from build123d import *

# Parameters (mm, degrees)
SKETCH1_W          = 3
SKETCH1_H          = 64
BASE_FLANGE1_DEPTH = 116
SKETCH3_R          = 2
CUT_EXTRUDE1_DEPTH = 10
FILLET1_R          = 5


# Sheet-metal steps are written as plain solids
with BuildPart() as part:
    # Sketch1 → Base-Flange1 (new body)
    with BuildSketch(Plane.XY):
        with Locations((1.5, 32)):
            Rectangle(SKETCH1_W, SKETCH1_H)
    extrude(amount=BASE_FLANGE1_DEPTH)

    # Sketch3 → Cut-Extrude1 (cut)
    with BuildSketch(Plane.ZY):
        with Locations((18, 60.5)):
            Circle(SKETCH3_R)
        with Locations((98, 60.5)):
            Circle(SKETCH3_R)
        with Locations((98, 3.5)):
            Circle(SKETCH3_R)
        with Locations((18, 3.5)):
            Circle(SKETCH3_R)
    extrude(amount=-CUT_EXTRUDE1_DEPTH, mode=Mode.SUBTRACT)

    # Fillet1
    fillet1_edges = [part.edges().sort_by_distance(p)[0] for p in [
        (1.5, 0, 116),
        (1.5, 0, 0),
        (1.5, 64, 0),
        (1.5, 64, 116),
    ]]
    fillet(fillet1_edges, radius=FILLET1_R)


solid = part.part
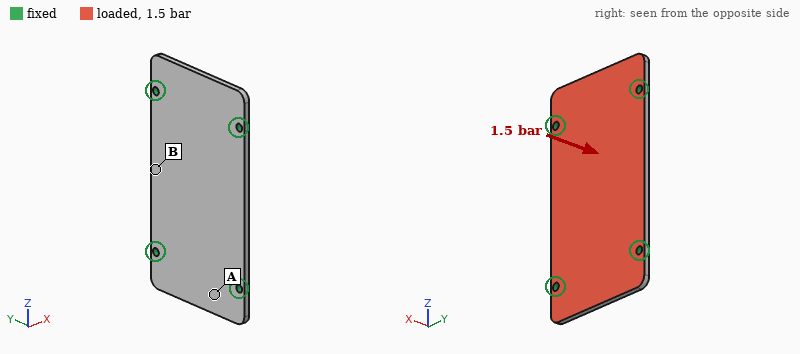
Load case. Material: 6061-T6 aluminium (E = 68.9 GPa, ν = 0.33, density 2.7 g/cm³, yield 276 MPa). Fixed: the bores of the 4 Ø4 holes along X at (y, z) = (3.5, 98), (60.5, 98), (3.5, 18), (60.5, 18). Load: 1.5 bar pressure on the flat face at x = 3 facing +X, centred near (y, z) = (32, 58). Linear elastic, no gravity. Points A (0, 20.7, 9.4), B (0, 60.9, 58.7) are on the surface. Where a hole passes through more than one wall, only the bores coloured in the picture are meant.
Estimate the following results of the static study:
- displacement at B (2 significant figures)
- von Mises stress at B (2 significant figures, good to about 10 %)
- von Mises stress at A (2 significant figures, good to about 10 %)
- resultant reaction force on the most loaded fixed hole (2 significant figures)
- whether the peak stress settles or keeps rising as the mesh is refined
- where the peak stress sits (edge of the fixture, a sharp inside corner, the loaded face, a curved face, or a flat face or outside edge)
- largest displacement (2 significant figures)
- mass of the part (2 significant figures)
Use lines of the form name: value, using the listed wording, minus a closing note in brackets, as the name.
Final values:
displacement at B: 0.13 mm
von Mises stress at B: 33 MPa
von Mises stress at A: 14 MPa
resultant reaction force on the most loaded fixed hole: 280 N
whether the peak stress settles or keeps rising as the mesh is refined: keeps rising
where the peak stress sits: edge of the fixture
largest displacement: 0.15 mm
mass of the part: 60 g
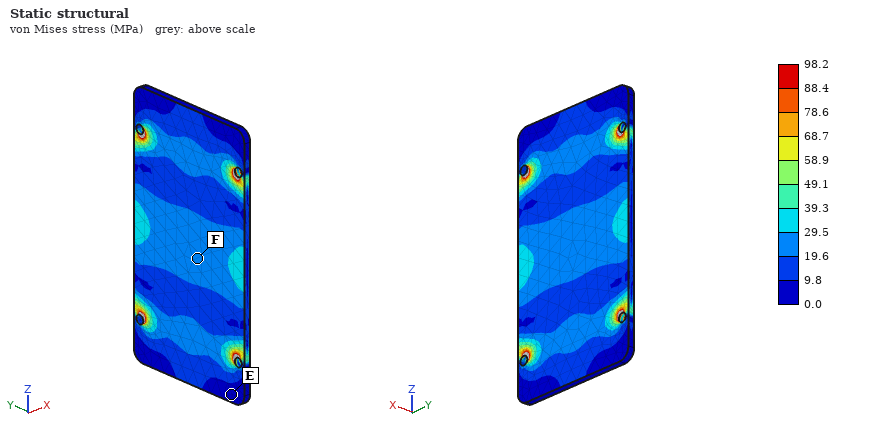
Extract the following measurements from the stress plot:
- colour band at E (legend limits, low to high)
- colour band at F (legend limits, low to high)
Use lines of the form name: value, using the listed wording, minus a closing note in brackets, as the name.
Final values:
colour band at E: 0.0 to 9.8 MPa
colour band at F: 19.6 to 29.5 MPa
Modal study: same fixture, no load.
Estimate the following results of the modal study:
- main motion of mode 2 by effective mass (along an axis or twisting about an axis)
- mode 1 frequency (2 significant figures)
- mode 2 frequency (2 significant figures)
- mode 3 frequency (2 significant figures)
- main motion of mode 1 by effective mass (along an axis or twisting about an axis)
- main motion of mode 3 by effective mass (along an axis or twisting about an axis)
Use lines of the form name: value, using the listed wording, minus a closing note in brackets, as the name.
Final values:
main motion of mode 2 by effective mass: twisting about Z
mode 1 frequency: 2000 Hz
mode 2 frequency: 3200 Hz
mode 3 frequency: 3900 Hz
main motion of mode 1 by effective mass: along X
main motion of mode 3 by effective mass: along X
